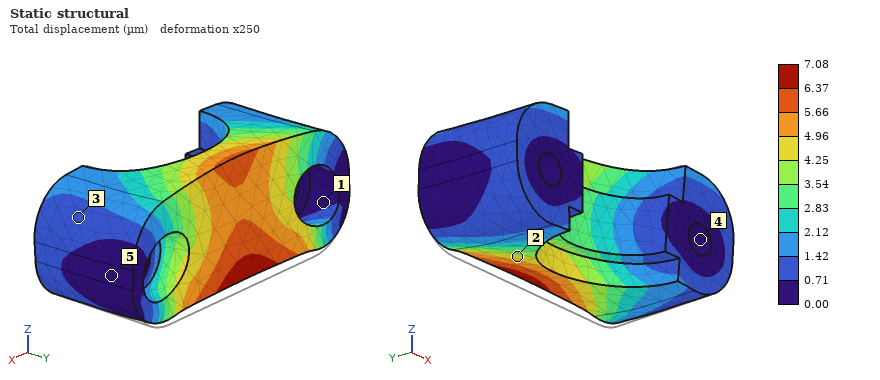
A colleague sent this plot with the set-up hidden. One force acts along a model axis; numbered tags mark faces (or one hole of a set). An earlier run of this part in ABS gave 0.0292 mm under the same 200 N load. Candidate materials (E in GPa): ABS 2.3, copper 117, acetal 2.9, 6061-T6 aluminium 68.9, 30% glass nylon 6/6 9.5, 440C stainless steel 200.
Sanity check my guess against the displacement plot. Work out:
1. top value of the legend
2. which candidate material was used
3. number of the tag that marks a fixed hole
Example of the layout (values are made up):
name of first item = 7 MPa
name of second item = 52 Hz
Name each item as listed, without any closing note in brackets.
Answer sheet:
top value of the legend = 7.08 µm
which candidate material was used = 30% glass nylon 6/6
number of the tag that marks a fixed hole = 4
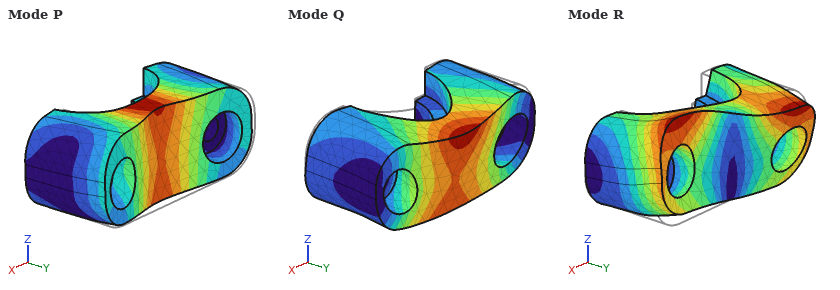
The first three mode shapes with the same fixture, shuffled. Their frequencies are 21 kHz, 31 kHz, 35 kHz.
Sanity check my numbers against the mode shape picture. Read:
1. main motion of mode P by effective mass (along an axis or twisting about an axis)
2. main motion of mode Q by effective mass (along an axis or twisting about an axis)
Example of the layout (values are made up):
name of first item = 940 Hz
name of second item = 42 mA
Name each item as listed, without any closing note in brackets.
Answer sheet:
main motion of mode P by effective mass = along Y
main motion of mode Q by effective mass = along Z
